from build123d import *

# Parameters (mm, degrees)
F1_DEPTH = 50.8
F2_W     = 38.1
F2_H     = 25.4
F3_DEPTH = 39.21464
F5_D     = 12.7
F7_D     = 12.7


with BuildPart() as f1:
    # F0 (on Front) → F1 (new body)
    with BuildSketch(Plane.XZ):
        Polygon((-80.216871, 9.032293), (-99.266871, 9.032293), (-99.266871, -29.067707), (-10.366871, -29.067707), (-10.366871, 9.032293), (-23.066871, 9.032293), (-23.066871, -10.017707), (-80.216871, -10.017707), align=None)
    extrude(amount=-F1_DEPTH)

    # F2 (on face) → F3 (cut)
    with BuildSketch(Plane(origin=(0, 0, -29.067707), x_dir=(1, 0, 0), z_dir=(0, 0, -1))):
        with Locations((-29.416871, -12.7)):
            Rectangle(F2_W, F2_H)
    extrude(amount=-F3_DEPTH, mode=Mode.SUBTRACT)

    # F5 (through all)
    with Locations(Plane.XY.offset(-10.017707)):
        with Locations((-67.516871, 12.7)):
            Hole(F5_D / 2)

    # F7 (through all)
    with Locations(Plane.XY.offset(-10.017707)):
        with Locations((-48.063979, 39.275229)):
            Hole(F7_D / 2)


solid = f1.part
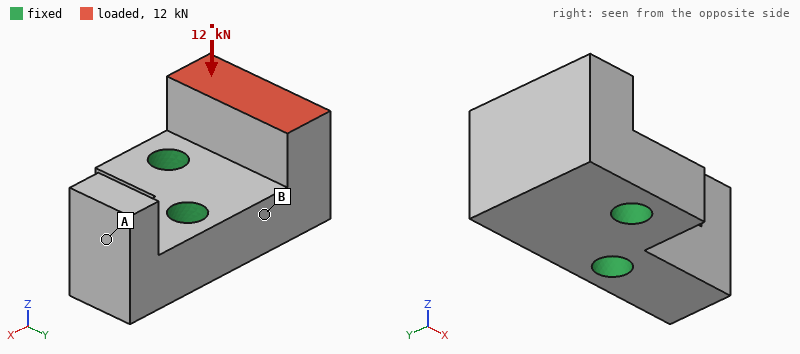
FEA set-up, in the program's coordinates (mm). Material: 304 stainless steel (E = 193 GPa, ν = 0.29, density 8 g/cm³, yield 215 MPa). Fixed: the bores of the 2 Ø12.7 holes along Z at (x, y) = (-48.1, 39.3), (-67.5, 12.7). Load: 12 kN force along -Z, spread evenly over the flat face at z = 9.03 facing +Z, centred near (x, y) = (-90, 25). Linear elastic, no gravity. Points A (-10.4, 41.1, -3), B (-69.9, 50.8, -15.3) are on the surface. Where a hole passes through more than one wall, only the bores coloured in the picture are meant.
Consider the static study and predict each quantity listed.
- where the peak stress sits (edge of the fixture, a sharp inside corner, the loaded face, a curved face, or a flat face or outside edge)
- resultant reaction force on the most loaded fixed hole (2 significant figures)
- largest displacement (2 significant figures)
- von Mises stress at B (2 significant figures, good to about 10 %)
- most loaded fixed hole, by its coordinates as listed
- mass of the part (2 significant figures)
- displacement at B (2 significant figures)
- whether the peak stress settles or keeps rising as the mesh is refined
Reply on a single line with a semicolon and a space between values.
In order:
edge of the fixture; 10 kN; 35 µm; 27 MPa; (-67.5, 12.7); 700 g; 6.7 µm; keeps rising
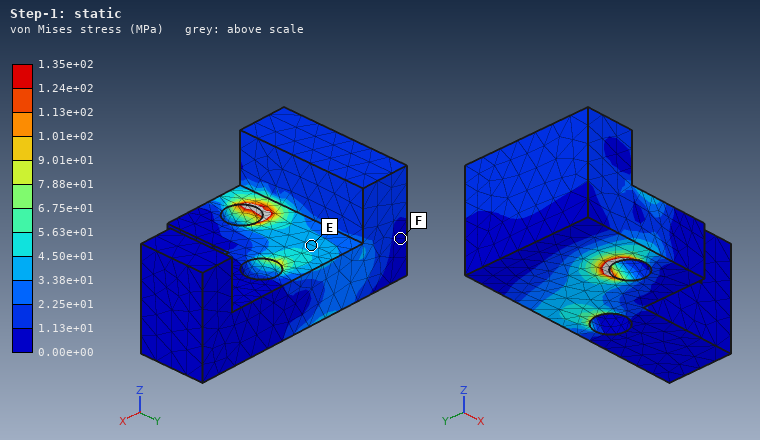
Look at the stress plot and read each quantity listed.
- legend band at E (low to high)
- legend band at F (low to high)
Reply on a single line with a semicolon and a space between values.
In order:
3.38e+01 to 4.50e+01 MPa; 0.00e+00 to 1.13e+01 MPa
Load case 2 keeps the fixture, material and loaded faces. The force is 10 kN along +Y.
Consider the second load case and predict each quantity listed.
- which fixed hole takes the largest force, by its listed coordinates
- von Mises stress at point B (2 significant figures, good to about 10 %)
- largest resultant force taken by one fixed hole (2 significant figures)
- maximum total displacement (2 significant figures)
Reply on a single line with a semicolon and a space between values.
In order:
(-67.5, 12.7); 54 MPa; 12 kN; 37 µm
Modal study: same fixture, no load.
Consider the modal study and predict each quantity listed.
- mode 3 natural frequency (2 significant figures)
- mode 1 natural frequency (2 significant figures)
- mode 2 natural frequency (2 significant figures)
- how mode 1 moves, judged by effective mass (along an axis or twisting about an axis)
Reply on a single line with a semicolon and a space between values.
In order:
7100 Hz; 6300 Hz; 6700 Hz; along Z
